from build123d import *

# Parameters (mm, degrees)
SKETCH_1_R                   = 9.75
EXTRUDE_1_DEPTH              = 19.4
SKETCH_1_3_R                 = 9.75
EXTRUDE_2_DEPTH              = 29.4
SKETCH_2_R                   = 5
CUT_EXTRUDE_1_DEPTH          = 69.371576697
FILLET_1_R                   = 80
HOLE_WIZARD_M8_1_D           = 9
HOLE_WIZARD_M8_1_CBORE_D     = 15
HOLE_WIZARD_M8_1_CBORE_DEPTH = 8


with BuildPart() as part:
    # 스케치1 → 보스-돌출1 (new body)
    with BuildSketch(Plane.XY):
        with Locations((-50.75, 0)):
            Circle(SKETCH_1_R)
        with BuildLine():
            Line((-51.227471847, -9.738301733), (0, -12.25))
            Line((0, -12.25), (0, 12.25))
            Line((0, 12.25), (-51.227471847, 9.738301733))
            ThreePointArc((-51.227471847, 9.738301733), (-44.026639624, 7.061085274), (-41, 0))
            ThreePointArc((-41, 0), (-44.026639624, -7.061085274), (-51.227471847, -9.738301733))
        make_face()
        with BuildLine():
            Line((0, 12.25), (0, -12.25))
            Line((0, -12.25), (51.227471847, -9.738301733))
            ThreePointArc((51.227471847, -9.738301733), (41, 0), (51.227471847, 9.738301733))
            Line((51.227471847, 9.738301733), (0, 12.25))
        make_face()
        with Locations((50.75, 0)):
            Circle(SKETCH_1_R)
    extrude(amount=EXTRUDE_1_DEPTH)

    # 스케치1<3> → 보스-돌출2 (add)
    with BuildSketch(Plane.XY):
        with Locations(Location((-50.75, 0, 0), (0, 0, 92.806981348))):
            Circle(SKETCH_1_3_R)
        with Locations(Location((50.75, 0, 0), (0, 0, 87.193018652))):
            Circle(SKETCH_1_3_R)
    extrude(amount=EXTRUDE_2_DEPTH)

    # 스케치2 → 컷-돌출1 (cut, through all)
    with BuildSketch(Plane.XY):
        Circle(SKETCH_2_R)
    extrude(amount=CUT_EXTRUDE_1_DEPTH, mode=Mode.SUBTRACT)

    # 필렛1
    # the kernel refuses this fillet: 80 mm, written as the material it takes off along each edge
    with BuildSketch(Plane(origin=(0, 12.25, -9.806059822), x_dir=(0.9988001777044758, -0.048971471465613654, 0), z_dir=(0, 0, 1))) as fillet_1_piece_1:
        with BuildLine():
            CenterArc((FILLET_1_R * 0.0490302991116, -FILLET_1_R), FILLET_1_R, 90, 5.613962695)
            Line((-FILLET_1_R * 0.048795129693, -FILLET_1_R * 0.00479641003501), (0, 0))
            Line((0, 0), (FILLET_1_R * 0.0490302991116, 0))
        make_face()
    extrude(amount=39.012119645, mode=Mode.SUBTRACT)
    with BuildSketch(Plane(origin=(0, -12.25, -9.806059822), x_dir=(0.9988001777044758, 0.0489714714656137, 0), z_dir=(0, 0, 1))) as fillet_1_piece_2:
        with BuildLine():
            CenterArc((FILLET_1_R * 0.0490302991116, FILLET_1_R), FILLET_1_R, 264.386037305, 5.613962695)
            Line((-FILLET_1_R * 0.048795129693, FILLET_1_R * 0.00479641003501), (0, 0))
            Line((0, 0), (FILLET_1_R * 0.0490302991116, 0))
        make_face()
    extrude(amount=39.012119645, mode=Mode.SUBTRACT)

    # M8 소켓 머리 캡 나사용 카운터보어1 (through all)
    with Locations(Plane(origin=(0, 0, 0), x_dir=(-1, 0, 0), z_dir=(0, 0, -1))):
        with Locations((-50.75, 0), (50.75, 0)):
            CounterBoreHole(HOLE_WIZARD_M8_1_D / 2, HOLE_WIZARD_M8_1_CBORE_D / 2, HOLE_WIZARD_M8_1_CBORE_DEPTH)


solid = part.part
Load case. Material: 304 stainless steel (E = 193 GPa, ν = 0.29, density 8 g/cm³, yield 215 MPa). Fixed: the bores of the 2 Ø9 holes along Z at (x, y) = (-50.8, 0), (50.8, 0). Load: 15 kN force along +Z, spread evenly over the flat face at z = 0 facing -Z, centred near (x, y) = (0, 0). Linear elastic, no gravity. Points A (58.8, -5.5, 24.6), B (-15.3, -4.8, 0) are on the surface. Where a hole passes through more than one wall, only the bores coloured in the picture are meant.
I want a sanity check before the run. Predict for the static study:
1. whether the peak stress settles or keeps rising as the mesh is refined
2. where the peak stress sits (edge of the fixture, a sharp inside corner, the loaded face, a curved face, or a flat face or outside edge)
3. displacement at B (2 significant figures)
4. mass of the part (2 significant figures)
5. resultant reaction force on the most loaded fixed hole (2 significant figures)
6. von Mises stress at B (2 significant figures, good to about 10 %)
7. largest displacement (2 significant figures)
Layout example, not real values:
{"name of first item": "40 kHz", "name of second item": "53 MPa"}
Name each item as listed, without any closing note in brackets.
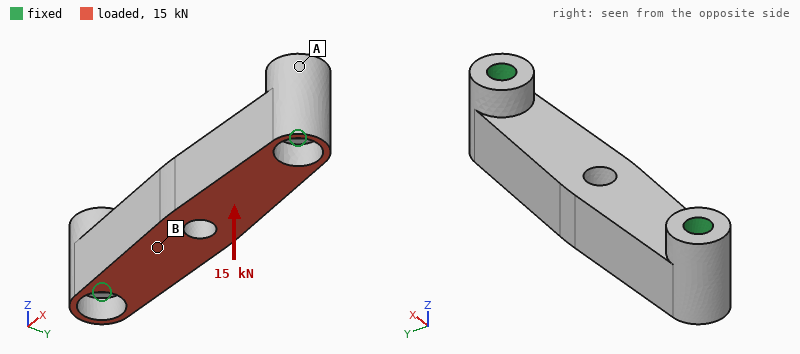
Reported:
{"whether the peak stress settles or keeps rising as the mesh is refined": "keeps rising", "where the peak stress sits": "edge of the fixture", "displacement at B": "25 µm", "mass of the part": "380 g", "resultant reaction force on the most loaded fixed hole": "8.5 kN", "von Mises stress at B": "43 MPa", "largest displacement": "30 µm"}
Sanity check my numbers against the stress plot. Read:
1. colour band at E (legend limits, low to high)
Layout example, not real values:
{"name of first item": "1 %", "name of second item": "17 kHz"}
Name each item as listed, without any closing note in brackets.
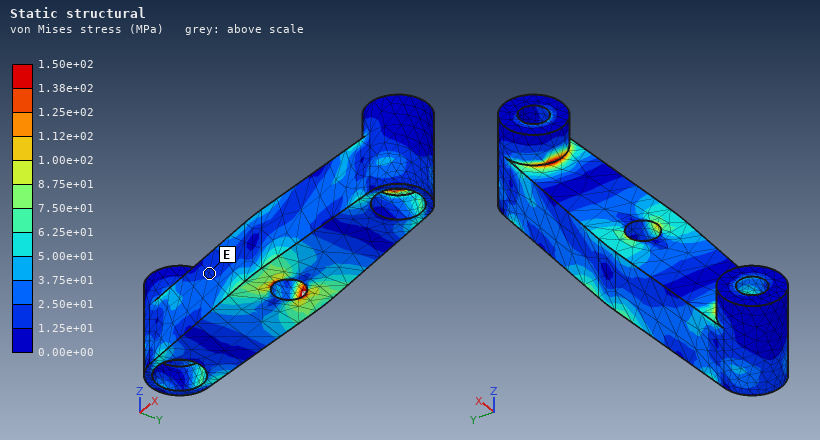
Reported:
{"colour band at E": "1.25e+01 to 2.50e+01 MPa"}
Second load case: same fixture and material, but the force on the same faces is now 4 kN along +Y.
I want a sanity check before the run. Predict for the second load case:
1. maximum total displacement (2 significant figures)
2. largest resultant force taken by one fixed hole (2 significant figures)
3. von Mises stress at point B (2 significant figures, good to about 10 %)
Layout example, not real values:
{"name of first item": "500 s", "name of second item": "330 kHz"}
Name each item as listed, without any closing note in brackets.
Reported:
{"maximum total displacement": "13 µm", "largest resultant force taken by one fixed hole": "2.0 kN", "von Mises stress at point B": "9.1 MPa"}
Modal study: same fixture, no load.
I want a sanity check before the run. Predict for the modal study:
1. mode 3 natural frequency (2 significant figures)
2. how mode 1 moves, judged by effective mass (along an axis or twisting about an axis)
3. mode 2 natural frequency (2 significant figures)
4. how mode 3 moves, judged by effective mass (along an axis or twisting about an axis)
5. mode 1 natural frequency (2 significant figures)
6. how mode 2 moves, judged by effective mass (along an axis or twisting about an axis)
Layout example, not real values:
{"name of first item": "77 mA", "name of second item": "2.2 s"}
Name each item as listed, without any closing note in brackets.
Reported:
{"mode 3 natural frequency": "12 kHz", "how mode 1 moves, judged by effective mass": "along Z", "mode 2 natural frequency": "7500 Hz", "how mode 3 moves, judged by effective mass": "twisting about X", "mode 1 natural frequency": "7100 Hz", "how mode 2 moves, judged by effective mass": "along Y"}
